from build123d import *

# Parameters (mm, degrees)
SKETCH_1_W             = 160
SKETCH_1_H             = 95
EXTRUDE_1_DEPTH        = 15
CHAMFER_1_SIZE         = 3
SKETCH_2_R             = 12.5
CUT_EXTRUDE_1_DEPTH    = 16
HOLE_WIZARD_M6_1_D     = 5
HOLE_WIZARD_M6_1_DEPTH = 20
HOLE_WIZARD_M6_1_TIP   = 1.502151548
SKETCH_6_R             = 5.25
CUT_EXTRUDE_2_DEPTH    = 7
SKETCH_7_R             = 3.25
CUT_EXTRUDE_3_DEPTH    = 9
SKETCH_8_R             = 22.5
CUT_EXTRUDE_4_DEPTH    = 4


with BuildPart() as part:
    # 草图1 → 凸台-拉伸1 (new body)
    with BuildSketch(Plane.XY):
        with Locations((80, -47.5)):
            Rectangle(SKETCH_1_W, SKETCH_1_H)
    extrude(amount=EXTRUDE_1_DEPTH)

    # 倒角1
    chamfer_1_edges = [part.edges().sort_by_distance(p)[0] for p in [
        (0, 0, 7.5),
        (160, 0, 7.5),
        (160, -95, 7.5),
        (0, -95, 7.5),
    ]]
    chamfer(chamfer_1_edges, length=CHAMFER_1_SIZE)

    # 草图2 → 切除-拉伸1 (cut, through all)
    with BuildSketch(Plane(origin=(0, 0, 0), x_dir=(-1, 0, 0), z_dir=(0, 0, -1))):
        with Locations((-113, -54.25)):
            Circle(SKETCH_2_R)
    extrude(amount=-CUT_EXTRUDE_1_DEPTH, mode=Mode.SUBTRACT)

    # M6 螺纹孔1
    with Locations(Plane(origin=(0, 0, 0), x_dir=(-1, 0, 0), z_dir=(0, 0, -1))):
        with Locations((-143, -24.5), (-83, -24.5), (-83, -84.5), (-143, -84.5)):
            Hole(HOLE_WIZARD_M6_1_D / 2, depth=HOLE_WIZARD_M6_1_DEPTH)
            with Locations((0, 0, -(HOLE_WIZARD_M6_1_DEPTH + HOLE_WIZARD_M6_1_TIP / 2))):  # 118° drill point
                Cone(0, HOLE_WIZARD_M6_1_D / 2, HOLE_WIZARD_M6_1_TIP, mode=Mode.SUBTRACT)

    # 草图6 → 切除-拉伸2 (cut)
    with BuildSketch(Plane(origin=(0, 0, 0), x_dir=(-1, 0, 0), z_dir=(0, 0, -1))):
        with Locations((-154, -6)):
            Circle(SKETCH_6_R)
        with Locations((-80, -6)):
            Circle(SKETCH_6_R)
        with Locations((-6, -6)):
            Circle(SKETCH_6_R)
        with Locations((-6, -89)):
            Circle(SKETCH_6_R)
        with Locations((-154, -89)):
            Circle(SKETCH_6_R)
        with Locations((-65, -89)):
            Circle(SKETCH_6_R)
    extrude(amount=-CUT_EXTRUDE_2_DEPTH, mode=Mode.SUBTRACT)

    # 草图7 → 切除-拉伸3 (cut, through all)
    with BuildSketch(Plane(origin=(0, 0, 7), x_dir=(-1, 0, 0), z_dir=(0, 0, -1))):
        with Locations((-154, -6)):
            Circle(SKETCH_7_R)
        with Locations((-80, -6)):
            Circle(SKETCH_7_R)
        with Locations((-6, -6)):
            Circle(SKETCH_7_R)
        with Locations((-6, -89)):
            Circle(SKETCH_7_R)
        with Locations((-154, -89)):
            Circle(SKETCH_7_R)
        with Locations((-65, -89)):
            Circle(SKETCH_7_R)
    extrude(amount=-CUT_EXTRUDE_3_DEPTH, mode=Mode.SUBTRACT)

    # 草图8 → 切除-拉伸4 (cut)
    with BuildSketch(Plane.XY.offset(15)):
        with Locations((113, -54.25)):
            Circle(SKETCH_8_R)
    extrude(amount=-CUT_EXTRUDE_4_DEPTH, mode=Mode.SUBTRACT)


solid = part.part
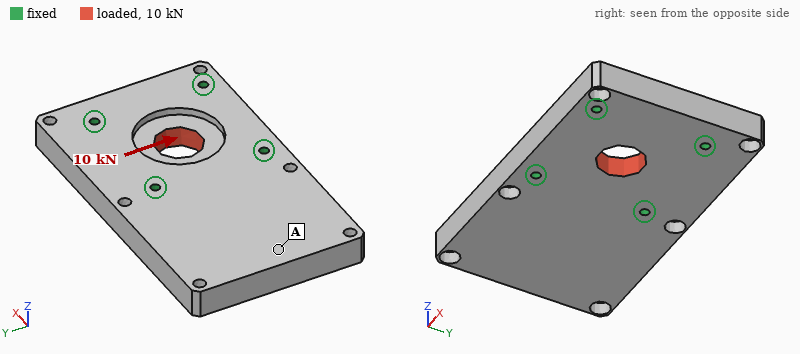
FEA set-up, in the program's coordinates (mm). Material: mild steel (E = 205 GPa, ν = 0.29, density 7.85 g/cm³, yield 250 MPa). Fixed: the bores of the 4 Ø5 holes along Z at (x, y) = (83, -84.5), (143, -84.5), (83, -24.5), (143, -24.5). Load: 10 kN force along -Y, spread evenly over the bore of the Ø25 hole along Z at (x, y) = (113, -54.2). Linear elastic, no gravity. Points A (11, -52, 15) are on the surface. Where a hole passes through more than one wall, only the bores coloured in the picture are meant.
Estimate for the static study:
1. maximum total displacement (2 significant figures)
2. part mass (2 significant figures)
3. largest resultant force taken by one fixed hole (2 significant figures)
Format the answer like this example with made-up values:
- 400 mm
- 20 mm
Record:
- 2.4 µm
- 1.6 kg
- 2.8 kN
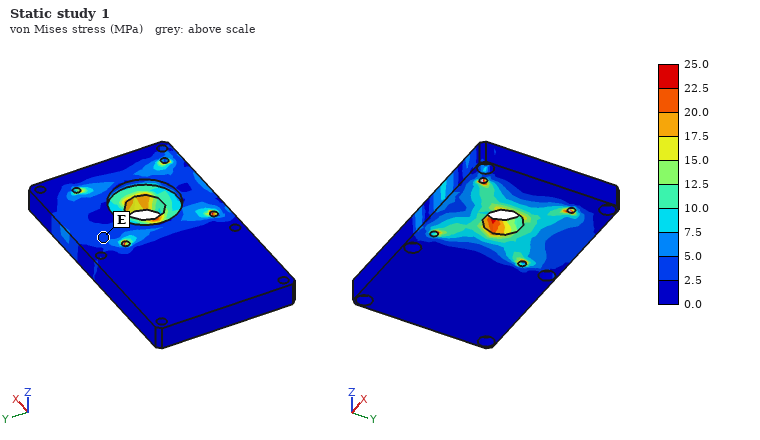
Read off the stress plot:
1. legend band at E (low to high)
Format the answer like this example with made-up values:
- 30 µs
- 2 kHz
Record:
- 2.5 to 5.0 MPa
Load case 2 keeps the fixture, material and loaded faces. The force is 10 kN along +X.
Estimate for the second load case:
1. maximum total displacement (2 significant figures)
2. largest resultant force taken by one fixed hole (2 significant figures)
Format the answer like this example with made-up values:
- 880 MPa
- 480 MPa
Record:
- 2.2 µm
- 2.7 kN
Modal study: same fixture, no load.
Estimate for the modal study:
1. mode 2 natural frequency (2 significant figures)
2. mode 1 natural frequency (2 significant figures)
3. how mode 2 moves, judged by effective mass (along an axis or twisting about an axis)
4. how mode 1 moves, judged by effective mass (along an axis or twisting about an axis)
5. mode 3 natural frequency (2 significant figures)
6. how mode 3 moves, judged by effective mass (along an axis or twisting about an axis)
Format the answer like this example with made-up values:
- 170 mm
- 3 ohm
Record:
- 3500 Hz
- 1500 Hz
- twisting about X
- along Z
- 5700 Hz
- along Y
